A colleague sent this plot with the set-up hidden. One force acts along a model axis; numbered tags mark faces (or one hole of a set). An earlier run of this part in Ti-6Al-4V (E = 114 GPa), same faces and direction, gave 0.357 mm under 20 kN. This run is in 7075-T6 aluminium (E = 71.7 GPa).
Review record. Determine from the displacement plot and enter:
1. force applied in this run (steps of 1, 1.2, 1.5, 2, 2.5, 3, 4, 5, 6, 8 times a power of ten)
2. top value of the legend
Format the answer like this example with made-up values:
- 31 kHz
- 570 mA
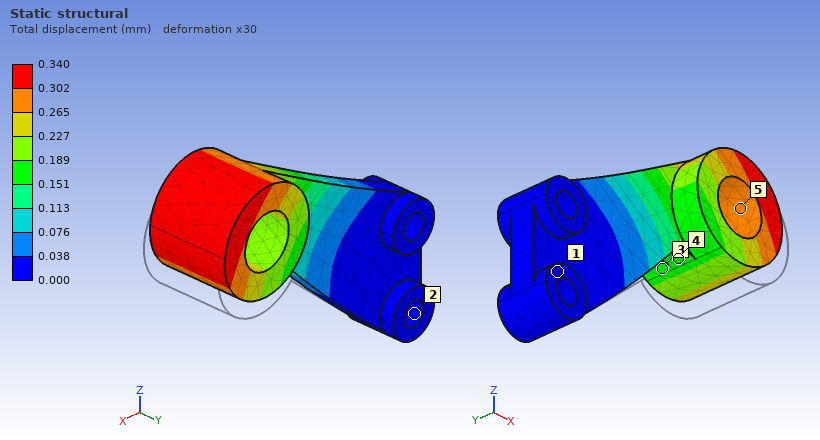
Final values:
- 12 kN
- 0.340 mm
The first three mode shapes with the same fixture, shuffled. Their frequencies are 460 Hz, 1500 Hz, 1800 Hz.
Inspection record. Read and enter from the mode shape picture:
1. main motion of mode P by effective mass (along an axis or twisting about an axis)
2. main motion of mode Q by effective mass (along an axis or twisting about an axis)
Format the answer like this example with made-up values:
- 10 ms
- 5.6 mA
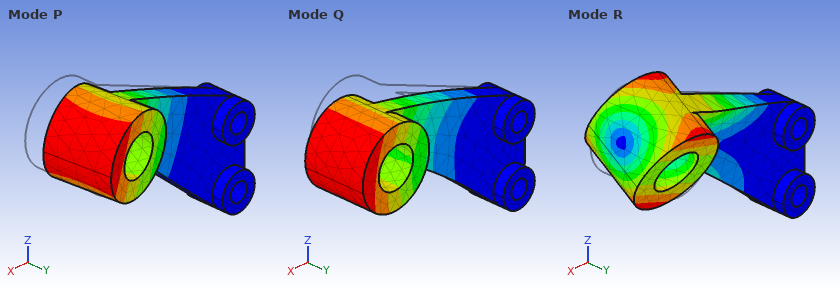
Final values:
- along Y
- along Z
